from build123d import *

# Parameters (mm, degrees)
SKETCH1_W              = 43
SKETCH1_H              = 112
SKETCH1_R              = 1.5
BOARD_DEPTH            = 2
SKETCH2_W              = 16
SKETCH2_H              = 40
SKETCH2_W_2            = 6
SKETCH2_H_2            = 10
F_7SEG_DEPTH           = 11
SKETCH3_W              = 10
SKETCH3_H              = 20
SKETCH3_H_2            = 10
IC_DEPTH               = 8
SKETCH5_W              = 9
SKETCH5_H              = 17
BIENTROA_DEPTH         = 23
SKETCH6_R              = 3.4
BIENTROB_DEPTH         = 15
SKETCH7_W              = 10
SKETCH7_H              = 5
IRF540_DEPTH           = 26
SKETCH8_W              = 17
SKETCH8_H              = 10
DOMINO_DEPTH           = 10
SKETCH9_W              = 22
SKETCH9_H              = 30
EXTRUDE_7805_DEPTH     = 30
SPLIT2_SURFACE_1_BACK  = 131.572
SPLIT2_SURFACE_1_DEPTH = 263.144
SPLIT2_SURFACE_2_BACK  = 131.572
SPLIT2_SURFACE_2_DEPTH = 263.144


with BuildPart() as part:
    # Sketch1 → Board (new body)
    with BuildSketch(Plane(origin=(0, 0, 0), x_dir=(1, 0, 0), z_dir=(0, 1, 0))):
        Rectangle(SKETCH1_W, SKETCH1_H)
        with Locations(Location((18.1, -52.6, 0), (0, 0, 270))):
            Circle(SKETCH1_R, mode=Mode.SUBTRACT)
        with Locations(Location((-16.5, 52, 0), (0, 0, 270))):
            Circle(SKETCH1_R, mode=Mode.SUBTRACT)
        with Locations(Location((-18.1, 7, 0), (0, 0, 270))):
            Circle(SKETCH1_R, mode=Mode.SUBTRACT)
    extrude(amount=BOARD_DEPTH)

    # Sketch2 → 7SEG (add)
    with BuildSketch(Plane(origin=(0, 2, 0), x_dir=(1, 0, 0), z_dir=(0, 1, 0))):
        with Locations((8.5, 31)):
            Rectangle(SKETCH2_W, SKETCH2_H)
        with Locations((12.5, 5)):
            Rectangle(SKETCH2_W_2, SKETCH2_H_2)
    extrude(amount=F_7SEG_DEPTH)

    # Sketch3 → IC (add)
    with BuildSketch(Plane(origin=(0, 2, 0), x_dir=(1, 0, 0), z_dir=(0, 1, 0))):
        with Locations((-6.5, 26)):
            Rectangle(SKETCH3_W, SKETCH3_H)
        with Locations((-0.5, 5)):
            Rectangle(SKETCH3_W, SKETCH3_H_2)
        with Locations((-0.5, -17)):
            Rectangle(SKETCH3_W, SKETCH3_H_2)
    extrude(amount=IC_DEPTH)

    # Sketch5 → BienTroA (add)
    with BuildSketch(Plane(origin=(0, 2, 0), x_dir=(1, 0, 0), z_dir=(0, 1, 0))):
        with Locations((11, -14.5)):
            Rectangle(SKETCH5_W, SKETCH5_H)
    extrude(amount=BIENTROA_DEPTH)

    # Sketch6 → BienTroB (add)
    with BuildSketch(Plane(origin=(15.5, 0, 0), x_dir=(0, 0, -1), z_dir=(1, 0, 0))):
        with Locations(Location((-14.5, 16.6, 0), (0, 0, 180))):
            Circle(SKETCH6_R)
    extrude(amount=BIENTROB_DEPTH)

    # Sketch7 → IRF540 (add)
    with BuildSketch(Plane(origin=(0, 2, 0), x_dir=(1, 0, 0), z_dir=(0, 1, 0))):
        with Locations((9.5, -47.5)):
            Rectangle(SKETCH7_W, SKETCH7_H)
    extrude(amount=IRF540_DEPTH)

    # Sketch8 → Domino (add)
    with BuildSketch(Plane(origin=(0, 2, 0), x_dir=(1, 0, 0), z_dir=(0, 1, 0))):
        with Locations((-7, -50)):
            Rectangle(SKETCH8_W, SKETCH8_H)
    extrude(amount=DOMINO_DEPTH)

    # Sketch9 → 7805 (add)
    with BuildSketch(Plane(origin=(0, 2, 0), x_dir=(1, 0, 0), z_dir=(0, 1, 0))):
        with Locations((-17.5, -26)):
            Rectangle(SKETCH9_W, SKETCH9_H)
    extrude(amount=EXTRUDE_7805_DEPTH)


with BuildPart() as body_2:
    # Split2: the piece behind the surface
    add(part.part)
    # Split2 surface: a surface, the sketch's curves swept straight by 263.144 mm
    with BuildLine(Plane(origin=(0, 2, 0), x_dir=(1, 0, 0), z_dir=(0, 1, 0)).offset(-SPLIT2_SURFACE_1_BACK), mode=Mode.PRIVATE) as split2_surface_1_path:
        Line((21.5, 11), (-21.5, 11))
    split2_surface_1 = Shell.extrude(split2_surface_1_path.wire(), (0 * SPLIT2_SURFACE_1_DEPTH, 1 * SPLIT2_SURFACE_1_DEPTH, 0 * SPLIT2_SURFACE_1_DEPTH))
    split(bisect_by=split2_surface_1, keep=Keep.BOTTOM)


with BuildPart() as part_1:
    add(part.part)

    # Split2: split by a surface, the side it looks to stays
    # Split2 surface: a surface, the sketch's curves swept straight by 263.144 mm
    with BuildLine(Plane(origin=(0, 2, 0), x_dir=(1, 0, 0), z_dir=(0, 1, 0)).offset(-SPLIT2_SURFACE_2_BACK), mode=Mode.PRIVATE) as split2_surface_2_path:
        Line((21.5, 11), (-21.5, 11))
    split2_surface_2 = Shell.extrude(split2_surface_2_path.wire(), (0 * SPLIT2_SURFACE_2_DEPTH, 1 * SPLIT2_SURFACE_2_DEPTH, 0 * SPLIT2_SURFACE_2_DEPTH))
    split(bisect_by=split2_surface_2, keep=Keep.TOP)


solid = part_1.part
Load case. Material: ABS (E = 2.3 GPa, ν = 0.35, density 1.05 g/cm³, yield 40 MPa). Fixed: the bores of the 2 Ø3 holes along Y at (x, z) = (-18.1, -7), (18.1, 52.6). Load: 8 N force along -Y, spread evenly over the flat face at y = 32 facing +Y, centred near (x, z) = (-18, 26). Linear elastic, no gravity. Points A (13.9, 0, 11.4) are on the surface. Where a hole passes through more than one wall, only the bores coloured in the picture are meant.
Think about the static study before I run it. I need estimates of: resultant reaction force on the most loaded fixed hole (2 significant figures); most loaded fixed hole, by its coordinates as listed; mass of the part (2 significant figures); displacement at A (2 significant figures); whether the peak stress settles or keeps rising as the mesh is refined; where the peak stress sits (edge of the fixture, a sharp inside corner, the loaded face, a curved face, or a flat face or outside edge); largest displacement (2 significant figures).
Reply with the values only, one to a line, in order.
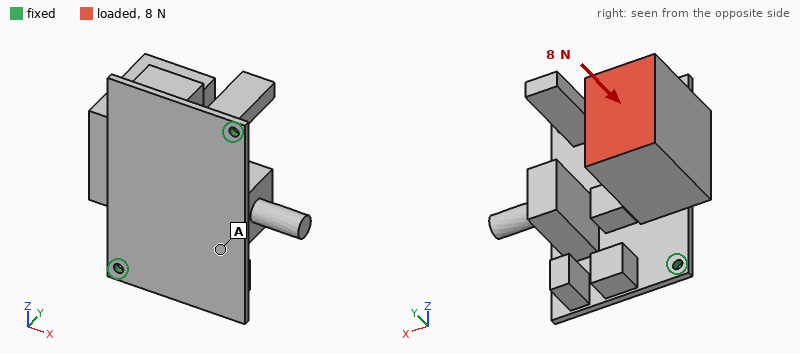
5.2 N
(-18.1, -7)
37 g
0.25 mm
keeps rising
edge of the fixture
0.98 mm
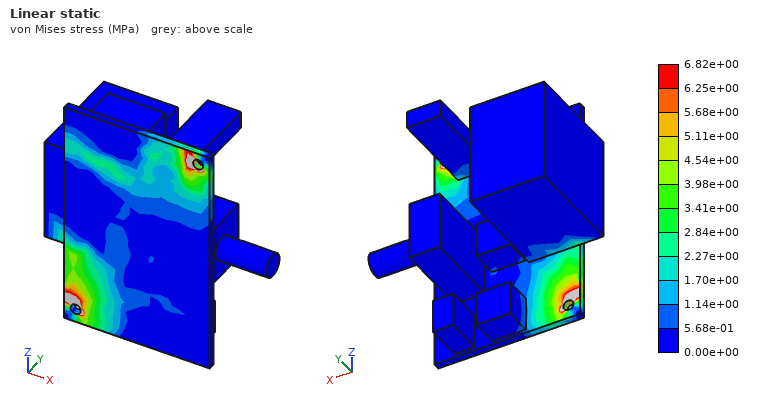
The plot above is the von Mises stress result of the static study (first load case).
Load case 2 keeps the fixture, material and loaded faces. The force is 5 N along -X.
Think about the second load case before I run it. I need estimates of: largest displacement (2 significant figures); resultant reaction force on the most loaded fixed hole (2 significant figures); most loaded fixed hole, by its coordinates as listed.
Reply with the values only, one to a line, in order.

1.0 mm
3.1 N
(18.1, 52.6)
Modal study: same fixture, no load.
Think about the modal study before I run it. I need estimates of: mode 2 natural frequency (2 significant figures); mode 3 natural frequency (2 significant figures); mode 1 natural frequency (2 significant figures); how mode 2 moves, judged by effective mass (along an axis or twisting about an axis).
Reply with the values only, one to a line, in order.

250 Hz
360 Hz
94 Hz
along Y
